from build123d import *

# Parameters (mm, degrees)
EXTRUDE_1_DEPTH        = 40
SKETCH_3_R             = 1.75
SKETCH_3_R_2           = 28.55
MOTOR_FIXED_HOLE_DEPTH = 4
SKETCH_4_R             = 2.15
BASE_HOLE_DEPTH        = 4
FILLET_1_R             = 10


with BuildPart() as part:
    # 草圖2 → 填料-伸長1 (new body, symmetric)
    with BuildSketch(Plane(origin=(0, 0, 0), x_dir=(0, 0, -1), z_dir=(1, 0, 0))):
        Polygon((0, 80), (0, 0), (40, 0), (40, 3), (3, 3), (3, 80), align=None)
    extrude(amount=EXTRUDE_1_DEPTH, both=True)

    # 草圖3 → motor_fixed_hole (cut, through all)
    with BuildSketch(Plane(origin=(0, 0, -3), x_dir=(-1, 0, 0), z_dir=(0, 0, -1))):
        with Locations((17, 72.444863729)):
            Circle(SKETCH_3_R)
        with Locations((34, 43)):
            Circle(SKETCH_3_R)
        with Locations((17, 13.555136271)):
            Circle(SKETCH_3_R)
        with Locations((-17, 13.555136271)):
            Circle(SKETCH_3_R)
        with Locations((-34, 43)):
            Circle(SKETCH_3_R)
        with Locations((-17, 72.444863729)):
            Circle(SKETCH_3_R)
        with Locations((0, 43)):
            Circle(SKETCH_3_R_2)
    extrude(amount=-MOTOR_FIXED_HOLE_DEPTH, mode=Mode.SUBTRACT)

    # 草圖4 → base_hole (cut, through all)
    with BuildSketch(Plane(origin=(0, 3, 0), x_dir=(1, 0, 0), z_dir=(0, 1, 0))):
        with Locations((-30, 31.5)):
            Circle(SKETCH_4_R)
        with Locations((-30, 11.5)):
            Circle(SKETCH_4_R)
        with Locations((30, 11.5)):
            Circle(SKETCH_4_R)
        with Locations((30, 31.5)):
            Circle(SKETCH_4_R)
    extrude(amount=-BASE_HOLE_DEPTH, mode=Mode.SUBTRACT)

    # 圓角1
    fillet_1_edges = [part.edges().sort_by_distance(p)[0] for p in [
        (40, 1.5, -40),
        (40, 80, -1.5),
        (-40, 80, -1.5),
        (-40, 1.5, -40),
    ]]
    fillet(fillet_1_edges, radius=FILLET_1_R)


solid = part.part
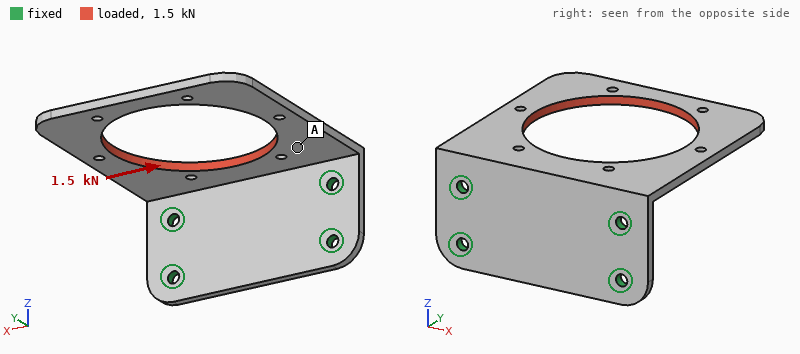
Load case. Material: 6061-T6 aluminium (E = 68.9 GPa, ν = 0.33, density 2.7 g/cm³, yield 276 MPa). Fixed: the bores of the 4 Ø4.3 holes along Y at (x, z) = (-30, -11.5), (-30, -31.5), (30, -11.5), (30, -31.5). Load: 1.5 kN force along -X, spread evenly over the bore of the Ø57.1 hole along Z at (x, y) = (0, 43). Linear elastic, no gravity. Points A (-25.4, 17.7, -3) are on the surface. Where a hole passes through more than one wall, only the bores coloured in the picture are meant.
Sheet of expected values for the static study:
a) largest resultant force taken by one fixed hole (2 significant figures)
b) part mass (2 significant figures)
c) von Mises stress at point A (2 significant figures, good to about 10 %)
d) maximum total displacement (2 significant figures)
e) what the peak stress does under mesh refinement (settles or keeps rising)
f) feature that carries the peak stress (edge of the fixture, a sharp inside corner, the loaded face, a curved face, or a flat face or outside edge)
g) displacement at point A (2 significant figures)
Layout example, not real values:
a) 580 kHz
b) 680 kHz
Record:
a) 1.2 kN
b) 53 g
c) 20 MPa
d) 0.47 mm
e) keeps rising
f) edge of the fixture
g) 0.12 mm
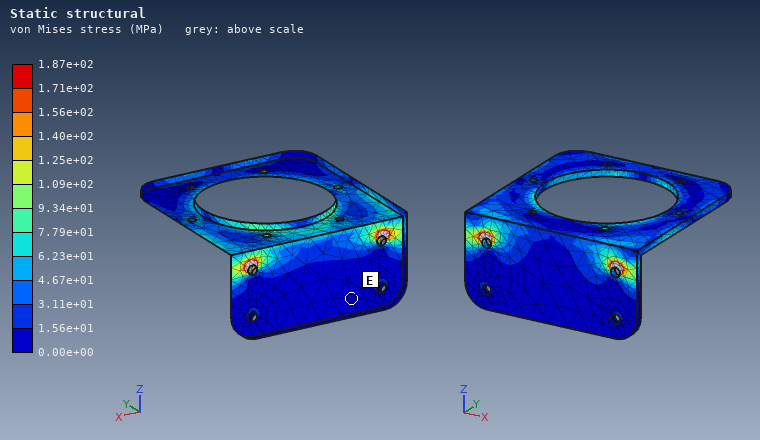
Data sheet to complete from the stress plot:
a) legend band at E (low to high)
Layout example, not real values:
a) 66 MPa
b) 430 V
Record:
a) 0.00e+00 to 1.56e+01 MPa
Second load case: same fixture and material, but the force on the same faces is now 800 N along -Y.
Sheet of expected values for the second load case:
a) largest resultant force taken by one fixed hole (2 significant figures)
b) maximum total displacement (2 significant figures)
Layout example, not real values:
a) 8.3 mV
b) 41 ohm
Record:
a) 450 N
b) 0.31 mm
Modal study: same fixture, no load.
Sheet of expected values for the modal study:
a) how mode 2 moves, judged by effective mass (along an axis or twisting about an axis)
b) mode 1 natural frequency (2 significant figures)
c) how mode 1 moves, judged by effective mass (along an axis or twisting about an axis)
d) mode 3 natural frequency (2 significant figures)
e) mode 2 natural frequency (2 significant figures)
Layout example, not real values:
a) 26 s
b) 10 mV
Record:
a) twisting about Y
b) 320 Hz
c) along Z
d) 1800 Hz
e) 720 Hz
